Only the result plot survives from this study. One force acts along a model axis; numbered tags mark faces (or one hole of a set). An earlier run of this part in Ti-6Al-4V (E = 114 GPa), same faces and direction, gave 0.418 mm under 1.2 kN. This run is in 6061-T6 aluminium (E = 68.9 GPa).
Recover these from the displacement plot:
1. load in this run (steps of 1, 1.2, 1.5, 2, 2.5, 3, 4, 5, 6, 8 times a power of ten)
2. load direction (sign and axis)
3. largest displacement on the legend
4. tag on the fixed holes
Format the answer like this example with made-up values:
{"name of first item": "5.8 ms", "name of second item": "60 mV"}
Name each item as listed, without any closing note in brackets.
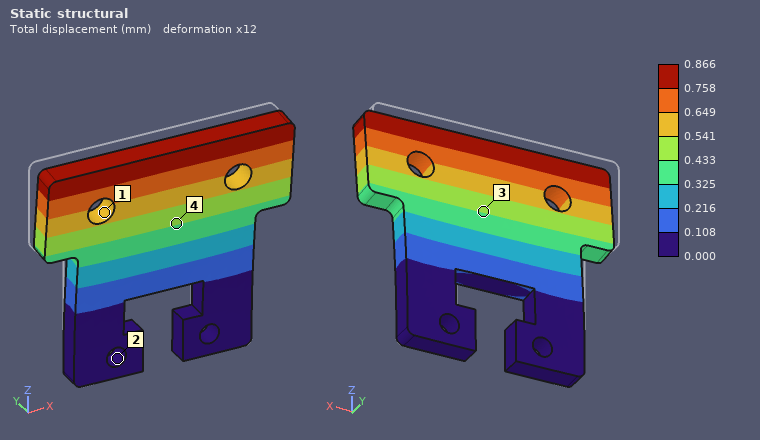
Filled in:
{"load in this run": "1.5 kN", "load direction": "-Y", "largest displacement on the legend": "0.866 mm", "tag on the fixed holes": "2"}
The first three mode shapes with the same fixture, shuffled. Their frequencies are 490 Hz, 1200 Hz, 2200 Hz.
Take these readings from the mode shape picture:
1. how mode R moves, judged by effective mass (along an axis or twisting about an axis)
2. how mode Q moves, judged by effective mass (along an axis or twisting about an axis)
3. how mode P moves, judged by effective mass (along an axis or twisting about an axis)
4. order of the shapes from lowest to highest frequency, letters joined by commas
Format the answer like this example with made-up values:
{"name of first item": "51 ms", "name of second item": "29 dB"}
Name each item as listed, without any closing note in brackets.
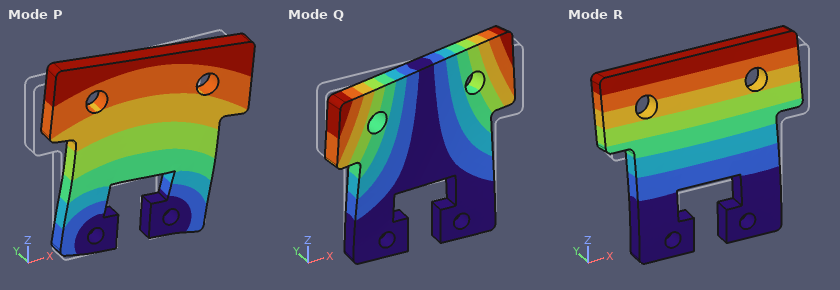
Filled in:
{"how mode R moves, judged by effective mass": "along Y", "how mode Q moves, judged by effective mass": "twisting about Z", "how mode P moves, judged by effective mass": "along X", "order of the shapes from lowest to highest frequency, letters joined by commas": "R, Q, P"}
